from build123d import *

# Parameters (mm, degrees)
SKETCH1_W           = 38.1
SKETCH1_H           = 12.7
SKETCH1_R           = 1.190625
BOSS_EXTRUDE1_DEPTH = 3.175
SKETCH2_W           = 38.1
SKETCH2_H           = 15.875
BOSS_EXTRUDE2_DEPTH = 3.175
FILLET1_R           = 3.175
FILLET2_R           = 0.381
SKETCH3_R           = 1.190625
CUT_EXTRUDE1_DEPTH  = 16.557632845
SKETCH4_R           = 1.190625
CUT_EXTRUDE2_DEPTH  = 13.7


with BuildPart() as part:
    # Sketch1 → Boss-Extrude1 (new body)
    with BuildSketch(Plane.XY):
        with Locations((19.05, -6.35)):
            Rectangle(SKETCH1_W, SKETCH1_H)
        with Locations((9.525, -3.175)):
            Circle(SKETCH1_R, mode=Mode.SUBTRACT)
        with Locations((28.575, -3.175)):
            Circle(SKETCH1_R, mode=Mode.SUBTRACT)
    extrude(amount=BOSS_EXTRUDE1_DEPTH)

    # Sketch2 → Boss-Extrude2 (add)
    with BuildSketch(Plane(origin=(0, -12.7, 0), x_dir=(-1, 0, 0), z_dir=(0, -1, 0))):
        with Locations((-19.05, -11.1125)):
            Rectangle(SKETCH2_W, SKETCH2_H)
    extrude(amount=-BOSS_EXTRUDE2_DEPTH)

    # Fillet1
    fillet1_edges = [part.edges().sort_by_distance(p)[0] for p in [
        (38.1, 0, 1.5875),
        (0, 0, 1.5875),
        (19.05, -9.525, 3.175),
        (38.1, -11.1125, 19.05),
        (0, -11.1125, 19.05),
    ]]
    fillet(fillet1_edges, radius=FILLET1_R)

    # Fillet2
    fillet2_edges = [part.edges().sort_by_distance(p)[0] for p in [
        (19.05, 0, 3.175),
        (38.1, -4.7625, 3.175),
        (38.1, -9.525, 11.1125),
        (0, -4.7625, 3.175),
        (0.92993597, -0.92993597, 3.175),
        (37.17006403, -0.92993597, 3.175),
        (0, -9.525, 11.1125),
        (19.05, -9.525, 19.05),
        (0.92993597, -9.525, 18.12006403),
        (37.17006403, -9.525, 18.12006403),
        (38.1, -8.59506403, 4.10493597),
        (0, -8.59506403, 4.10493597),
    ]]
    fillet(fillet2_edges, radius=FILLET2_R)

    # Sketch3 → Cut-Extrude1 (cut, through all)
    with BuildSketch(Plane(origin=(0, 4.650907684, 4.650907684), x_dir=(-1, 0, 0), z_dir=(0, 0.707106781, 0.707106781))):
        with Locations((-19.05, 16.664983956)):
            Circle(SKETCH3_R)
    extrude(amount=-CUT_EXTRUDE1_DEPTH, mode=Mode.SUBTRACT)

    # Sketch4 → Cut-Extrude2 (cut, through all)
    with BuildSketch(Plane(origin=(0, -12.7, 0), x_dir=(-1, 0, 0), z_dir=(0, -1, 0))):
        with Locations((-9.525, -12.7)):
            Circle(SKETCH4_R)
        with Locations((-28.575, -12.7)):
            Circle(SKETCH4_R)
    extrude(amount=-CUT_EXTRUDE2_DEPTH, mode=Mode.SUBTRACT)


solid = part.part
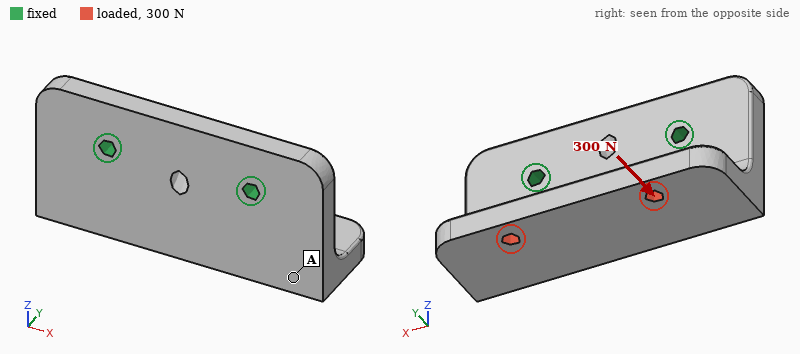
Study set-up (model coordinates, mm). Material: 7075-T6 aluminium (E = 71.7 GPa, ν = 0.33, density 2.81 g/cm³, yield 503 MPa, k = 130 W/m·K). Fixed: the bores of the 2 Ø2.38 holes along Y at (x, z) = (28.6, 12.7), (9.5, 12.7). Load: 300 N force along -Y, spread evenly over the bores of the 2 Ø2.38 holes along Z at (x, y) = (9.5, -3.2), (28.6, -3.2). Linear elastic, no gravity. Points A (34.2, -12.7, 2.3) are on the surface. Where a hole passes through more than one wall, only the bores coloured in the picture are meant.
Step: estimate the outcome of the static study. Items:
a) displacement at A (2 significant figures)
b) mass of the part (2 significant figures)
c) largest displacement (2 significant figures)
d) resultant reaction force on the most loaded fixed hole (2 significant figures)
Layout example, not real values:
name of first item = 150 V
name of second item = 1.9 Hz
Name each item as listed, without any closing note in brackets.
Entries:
displacement at A = 24 µm
mass of the part = 9.6 g
largest displacement = 45 µm
resultant reaction force on the most loaded fixed hole = 150 N
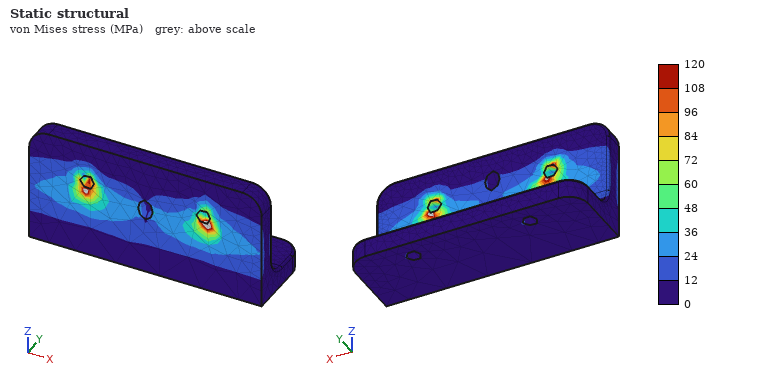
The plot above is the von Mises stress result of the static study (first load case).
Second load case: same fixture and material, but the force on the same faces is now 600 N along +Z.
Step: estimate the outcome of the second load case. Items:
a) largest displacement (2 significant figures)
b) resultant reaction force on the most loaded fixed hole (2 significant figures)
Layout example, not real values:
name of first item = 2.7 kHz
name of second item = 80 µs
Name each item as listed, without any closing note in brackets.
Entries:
largest displacement = 0.10 mm
resultant reaction force on the most loaded fixed hole = 300 N
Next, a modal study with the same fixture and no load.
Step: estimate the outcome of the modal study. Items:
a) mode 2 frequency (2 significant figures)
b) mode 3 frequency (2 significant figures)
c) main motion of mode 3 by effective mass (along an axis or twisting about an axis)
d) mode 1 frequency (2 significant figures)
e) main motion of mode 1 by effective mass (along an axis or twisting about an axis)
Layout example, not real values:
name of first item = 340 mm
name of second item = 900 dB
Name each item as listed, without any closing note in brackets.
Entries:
mode 2 frequency = 9600 Hz
mode 3 frequency = 21 kHz
main motion of mode 3 by effective mass = along X
mode 1 frequency = 6400 Hz
main motion of mode 1 by effective mass = along Y
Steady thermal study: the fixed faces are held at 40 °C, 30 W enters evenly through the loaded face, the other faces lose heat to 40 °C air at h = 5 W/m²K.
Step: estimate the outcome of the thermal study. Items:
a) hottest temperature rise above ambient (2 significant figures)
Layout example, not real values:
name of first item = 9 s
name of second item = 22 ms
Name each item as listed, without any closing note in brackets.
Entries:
hottest temperature rise above ambient = 45 K
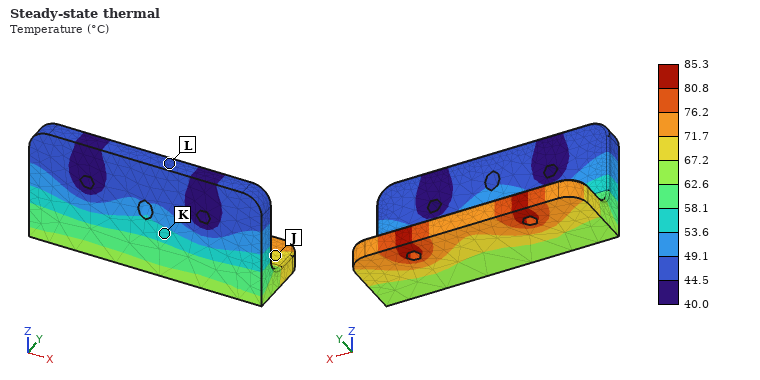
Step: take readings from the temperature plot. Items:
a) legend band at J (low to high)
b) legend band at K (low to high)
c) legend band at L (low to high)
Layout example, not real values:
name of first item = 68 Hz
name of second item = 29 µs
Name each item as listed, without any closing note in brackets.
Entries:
legend band at J = 67.2 to 71.7 °C
legend band at K = 53.6 to 58.1 °C
legend band at L = 44.5 to 49.1 °C
